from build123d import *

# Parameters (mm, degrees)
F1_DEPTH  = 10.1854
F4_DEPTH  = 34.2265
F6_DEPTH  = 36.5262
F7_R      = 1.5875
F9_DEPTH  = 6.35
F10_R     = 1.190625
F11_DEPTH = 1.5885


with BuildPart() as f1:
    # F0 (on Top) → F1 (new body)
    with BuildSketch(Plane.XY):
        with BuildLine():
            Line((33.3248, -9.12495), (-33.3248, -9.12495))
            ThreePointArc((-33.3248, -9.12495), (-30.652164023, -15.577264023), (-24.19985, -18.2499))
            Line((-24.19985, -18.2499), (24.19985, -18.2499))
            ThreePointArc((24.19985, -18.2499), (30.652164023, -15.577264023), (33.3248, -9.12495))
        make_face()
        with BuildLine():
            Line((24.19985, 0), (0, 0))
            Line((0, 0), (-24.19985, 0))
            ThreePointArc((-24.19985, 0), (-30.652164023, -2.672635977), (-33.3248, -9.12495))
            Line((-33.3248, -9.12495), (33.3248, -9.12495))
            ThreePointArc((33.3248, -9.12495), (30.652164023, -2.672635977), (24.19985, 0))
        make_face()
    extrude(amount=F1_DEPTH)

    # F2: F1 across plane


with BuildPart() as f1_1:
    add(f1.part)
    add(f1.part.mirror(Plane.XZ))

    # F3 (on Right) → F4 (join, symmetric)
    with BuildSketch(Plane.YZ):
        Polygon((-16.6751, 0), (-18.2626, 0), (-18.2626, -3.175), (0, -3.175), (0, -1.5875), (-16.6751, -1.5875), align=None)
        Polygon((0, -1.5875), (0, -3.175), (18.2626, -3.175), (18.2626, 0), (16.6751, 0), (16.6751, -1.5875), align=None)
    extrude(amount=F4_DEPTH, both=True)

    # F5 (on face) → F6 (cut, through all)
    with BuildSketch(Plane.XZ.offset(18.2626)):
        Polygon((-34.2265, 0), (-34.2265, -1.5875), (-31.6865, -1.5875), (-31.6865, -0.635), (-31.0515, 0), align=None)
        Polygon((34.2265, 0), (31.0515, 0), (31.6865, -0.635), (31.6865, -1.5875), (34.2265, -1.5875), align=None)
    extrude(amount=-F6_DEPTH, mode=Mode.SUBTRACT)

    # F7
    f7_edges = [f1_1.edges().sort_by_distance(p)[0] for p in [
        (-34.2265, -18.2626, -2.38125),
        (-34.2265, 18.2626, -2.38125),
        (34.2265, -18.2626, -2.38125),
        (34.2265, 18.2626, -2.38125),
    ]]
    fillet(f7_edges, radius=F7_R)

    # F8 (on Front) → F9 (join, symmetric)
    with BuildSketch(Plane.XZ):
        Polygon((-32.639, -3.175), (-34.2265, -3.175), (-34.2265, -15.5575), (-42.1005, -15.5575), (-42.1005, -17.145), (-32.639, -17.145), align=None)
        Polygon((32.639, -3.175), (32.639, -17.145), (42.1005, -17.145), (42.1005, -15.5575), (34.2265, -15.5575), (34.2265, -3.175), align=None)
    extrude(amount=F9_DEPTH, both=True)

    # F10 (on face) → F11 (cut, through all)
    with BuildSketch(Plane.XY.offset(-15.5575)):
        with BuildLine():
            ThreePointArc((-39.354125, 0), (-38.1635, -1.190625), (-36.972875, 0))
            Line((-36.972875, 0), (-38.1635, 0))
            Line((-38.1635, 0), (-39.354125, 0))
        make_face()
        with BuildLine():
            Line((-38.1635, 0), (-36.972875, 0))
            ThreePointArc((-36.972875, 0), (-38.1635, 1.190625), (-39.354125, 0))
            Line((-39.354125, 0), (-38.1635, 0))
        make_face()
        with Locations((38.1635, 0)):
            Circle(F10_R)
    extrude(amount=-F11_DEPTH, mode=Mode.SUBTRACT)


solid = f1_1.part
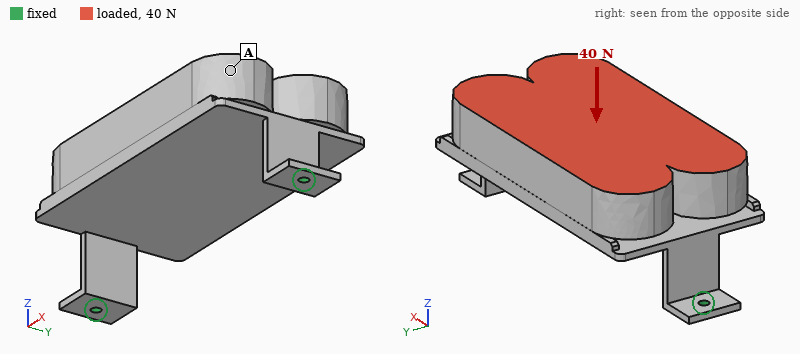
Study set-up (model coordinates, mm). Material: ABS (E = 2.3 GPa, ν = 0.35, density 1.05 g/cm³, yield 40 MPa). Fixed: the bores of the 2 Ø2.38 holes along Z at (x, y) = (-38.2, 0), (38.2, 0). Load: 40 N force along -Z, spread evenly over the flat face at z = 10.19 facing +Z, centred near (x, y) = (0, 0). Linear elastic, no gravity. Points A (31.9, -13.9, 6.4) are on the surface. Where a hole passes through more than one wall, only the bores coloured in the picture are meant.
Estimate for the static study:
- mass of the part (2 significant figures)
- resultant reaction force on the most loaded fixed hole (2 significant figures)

30 g
21 N
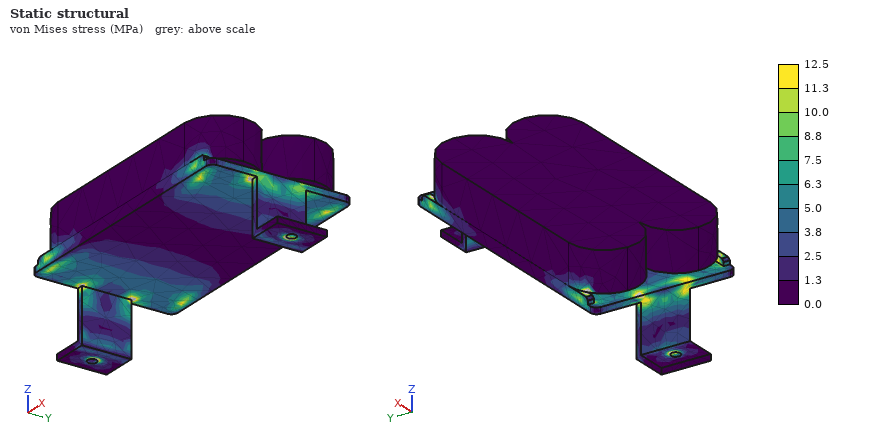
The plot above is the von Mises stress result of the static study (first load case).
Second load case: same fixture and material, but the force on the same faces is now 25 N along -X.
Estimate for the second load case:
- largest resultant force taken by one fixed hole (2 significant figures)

15 N
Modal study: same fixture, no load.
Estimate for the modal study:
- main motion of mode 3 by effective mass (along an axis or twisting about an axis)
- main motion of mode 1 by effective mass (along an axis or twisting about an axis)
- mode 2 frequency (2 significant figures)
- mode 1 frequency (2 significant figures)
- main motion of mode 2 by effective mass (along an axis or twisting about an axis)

along Z
along Y
190 Hz
110 Hz
along X
